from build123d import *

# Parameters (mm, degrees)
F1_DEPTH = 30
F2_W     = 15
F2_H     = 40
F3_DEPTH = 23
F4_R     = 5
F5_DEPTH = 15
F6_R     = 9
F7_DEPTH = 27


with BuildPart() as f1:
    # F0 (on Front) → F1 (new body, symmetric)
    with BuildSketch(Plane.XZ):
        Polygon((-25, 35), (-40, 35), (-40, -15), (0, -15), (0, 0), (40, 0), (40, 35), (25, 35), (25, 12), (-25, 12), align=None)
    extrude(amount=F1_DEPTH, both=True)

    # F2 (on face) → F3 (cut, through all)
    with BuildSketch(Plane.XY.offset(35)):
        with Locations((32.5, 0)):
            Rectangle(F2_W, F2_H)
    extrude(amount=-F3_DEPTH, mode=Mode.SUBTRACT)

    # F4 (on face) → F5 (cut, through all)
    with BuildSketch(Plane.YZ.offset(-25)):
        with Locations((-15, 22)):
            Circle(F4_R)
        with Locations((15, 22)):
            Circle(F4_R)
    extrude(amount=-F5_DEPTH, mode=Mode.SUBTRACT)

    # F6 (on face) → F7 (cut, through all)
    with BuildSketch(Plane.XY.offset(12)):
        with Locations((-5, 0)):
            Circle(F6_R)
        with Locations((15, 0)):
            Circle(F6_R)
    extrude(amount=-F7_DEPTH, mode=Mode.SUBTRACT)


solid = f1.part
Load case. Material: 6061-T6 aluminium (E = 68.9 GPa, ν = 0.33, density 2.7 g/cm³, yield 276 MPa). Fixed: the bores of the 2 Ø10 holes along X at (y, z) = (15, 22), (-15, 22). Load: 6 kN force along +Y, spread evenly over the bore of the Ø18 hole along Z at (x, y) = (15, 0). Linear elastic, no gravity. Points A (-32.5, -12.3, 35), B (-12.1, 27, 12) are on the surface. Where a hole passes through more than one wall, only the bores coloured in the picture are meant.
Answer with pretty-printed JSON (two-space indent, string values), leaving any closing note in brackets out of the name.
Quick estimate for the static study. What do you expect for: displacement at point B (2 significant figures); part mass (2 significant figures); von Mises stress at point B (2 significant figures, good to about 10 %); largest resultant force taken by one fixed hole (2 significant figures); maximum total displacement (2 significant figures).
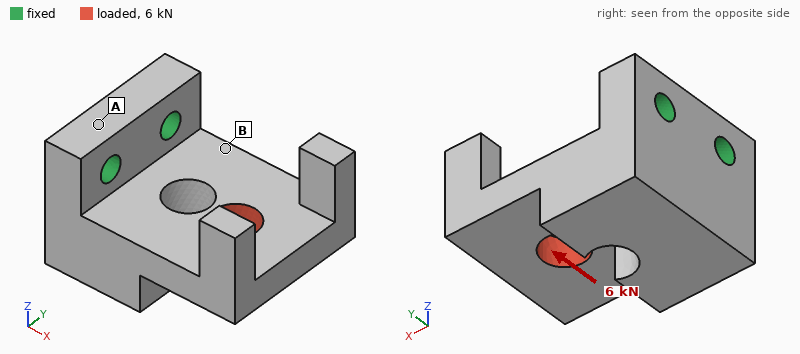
{
  "displacement at point B": "0.043 mm",
  "part mass": "300 g",
  "von Mises stress at point B": "31 MPa",
  "largest resultant force taken by one fixed hole": "7.5 kN",
  "maximum total displacement": "0.14 mm"
}
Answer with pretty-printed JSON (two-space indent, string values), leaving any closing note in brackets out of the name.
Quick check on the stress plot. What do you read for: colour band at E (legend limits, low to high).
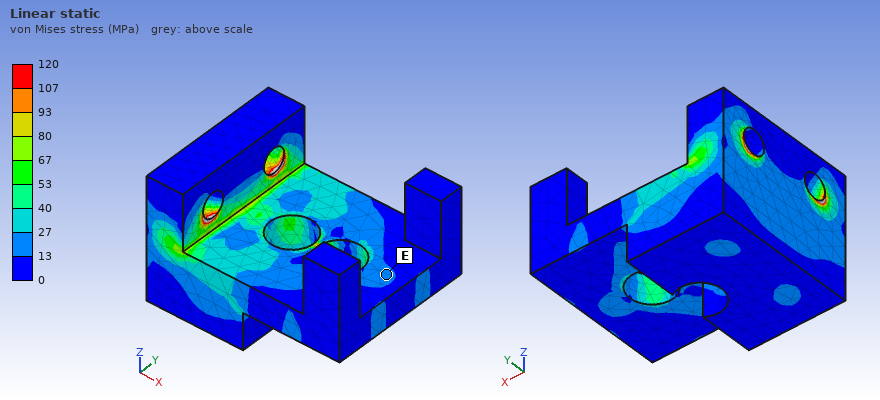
{
  "colour band at E": "13 to 27 MPa"
}
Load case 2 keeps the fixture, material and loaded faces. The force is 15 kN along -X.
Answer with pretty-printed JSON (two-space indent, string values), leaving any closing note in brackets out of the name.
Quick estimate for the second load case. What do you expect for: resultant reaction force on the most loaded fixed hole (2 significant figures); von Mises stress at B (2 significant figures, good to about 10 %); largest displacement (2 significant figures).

{
  "resultant reaction force on the most loaded fixed hole": "7.5 kN",
  "von Mises stress at B": "27 MPa",
  "largest displacement": "97 µm"
}
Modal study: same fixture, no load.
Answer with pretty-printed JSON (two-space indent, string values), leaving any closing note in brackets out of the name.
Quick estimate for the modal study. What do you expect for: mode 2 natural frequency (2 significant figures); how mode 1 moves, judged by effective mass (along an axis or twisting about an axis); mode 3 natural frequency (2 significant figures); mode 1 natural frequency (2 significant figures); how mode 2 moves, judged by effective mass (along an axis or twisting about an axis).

{
  "mode 2 natural frequency": "3200 Hz",
  "how mode 1 moves, judged by effective mass": "along Z",
  "mode 3 natural frequency": "4300 Hz",
  "mode 1 natural frequency": "1800 Hz",
  "how mode 2 moves, judged by effective mass": "along Y"
}
